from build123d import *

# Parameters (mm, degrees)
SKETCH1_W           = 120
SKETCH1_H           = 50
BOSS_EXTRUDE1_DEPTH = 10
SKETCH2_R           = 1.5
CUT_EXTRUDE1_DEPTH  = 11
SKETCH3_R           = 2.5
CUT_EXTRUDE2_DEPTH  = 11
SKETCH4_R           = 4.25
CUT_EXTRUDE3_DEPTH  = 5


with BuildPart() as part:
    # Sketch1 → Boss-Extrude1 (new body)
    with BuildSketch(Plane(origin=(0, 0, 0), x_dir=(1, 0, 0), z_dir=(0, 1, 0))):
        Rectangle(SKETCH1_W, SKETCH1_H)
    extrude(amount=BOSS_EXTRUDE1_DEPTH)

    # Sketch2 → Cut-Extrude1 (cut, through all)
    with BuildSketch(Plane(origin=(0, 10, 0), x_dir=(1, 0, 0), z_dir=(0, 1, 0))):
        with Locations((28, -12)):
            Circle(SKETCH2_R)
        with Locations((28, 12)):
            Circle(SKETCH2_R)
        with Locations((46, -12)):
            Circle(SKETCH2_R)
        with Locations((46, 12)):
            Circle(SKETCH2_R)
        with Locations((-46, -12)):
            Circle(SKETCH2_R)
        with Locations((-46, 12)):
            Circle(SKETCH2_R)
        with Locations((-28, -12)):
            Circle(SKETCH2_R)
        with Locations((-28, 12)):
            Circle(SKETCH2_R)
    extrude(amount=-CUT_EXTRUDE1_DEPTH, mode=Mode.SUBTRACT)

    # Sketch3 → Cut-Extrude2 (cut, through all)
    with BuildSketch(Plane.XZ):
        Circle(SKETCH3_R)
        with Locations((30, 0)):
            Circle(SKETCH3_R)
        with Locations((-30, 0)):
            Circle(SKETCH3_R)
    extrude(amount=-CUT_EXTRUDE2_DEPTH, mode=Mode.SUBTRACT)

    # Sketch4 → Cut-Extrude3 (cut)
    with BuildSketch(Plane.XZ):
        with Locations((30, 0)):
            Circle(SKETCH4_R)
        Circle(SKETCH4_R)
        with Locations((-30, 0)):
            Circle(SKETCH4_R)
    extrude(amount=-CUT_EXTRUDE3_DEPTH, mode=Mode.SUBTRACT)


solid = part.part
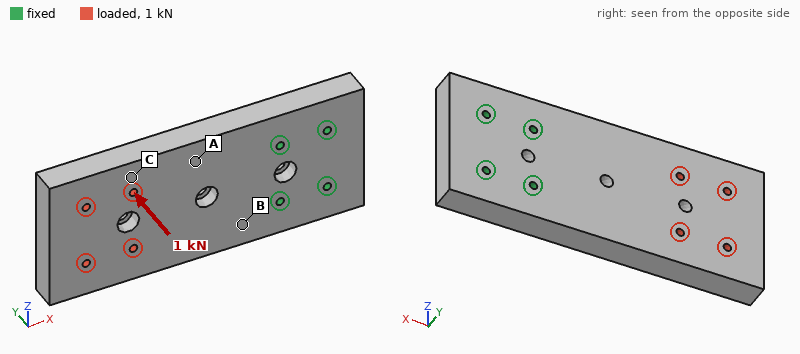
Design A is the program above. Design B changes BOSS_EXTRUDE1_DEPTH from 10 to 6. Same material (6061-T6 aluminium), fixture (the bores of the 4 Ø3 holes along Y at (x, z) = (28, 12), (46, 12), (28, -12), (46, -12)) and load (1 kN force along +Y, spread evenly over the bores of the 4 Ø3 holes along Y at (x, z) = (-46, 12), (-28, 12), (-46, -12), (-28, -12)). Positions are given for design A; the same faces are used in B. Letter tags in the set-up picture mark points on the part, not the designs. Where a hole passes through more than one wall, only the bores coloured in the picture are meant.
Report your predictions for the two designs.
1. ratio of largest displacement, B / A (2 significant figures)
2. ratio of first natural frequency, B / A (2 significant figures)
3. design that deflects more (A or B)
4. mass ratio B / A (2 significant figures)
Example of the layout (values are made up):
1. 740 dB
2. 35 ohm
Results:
1. 4.4
2. 0.62
3. B
4. 0.60
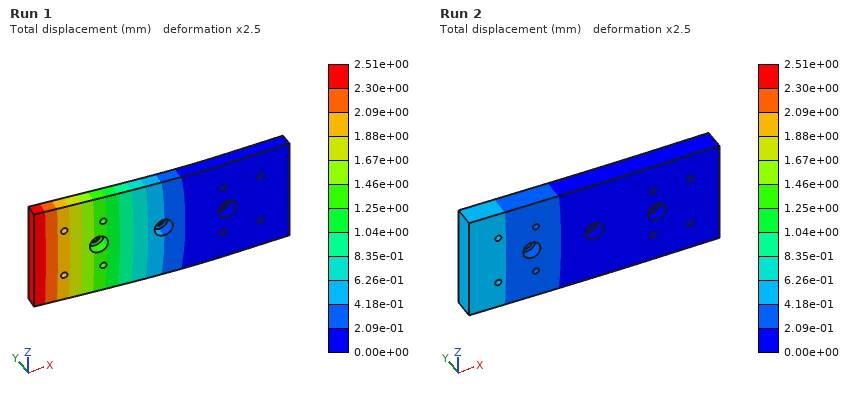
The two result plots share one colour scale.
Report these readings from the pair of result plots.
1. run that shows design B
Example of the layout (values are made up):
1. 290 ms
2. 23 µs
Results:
1. Run 1
